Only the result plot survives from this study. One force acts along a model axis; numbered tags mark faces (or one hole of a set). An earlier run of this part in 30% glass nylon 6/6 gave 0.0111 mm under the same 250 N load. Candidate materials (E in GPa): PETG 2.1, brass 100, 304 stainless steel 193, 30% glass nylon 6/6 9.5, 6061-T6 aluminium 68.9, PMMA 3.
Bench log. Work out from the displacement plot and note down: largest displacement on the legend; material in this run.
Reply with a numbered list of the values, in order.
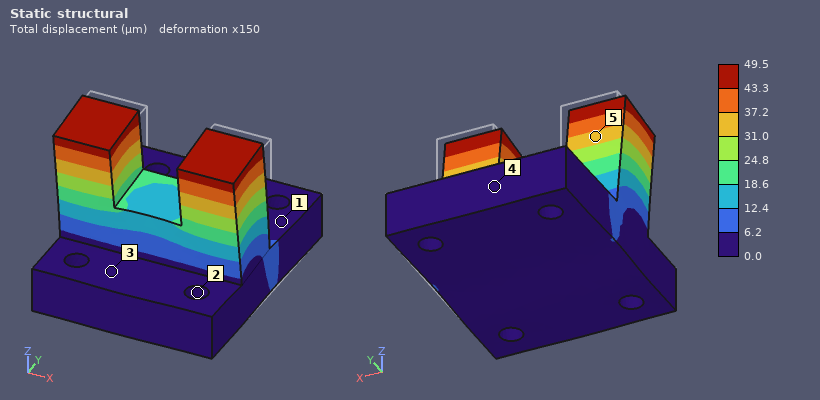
1. 49.5 µm
2. PETG
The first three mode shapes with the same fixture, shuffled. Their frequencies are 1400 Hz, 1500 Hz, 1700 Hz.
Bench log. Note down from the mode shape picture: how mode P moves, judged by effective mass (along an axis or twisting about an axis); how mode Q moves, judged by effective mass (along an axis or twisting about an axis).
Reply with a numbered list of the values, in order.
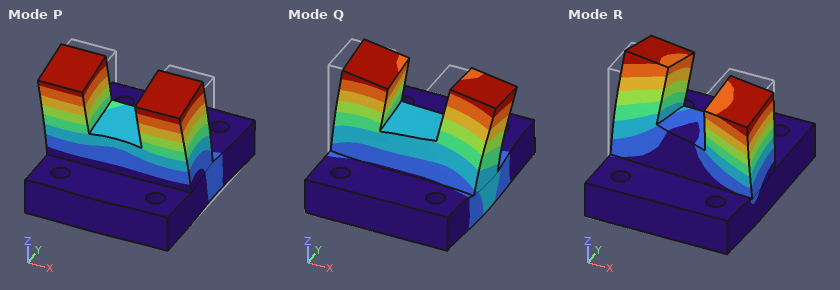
1. along Y
2. along X
